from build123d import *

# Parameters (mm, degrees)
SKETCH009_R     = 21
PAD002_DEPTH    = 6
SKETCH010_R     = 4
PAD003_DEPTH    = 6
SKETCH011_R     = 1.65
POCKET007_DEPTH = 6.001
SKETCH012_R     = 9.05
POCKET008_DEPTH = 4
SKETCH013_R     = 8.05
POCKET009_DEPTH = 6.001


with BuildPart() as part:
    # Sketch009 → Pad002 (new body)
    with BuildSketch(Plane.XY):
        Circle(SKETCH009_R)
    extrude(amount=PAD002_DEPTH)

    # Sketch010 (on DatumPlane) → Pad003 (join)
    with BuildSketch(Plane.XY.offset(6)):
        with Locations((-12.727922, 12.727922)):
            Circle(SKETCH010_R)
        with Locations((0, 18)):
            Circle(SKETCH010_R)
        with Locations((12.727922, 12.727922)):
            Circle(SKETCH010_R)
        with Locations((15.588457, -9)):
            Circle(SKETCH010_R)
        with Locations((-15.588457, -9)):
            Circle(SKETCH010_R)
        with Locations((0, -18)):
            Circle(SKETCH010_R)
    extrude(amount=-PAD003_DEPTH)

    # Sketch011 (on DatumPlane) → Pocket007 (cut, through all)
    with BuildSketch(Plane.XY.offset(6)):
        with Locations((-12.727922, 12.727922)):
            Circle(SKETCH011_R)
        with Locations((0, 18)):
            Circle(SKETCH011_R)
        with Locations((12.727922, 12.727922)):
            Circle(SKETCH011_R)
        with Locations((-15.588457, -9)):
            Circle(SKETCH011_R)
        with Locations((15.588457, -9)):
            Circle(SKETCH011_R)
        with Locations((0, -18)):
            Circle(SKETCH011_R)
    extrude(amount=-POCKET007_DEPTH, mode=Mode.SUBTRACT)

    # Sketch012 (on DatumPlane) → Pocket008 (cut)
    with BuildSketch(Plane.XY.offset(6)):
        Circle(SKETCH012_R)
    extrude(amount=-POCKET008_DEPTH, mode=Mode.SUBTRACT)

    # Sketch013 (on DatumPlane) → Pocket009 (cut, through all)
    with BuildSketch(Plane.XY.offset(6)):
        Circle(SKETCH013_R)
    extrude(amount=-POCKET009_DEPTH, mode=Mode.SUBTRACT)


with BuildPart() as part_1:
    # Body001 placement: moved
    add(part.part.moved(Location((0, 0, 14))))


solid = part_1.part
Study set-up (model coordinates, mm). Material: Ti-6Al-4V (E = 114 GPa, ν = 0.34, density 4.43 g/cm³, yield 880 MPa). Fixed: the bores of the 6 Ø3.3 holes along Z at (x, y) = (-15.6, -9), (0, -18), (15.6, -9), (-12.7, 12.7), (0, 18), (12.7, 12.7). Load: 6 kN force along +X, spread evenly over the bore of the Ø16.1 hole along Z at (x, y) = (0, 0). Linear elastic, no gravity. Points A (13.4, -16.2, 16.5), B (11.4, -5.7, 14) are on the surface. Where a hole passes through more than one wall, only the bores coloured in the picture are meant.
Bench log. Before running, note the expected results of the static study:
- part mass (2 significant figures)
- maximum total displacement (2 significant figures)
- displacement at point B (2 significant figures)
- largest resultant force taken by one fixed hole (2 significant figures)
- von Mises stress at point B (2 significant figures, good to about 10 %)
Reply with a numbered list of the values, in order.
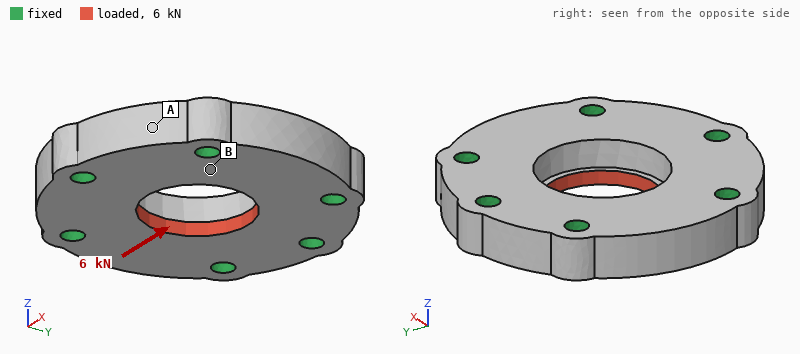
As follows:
1. 30 g
2. 6.8 µm
3. 2.2 µm
4. 1.4 kN
5. 54 MPa
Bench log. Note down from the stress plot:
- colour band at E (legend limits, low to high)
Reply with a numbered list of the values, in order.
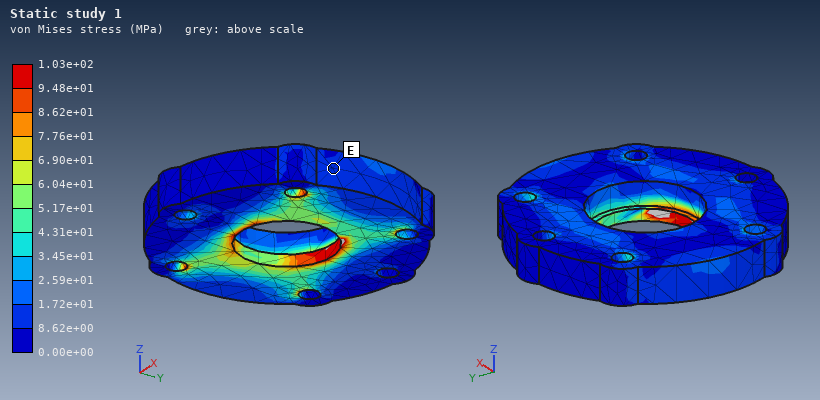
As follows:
1. 8.62e+00 to 1.72e+01 MPa
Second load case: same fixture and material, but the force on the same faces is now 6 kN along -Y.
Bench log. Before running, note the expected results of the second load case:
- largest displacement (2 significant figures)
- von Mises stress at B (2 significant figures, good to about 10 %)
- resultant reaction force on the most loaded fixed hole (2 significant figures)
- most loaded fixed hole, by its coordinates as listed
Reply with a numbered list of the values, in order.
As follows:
1. 5.6 µm
2. 26 MPa
3. 1.5 kN
4. (0, -18)
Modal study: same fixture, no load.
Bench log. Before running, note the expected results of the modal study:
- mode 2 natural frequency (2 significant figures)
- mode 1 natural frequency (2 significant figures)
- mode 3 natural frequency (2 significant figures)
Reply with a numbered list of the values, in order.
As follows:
1. 45 kHz
2. 44 kHz
3. 47 kHz
